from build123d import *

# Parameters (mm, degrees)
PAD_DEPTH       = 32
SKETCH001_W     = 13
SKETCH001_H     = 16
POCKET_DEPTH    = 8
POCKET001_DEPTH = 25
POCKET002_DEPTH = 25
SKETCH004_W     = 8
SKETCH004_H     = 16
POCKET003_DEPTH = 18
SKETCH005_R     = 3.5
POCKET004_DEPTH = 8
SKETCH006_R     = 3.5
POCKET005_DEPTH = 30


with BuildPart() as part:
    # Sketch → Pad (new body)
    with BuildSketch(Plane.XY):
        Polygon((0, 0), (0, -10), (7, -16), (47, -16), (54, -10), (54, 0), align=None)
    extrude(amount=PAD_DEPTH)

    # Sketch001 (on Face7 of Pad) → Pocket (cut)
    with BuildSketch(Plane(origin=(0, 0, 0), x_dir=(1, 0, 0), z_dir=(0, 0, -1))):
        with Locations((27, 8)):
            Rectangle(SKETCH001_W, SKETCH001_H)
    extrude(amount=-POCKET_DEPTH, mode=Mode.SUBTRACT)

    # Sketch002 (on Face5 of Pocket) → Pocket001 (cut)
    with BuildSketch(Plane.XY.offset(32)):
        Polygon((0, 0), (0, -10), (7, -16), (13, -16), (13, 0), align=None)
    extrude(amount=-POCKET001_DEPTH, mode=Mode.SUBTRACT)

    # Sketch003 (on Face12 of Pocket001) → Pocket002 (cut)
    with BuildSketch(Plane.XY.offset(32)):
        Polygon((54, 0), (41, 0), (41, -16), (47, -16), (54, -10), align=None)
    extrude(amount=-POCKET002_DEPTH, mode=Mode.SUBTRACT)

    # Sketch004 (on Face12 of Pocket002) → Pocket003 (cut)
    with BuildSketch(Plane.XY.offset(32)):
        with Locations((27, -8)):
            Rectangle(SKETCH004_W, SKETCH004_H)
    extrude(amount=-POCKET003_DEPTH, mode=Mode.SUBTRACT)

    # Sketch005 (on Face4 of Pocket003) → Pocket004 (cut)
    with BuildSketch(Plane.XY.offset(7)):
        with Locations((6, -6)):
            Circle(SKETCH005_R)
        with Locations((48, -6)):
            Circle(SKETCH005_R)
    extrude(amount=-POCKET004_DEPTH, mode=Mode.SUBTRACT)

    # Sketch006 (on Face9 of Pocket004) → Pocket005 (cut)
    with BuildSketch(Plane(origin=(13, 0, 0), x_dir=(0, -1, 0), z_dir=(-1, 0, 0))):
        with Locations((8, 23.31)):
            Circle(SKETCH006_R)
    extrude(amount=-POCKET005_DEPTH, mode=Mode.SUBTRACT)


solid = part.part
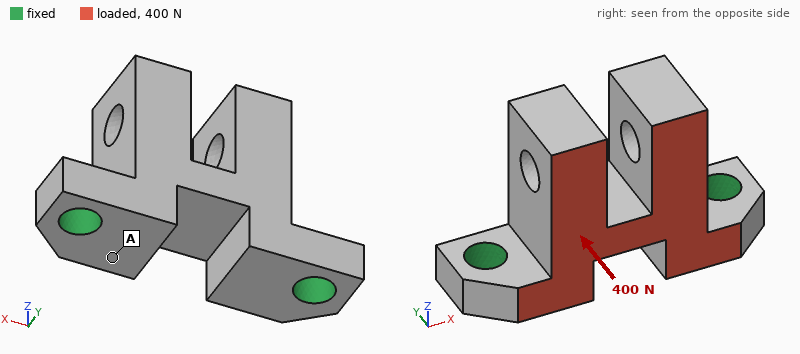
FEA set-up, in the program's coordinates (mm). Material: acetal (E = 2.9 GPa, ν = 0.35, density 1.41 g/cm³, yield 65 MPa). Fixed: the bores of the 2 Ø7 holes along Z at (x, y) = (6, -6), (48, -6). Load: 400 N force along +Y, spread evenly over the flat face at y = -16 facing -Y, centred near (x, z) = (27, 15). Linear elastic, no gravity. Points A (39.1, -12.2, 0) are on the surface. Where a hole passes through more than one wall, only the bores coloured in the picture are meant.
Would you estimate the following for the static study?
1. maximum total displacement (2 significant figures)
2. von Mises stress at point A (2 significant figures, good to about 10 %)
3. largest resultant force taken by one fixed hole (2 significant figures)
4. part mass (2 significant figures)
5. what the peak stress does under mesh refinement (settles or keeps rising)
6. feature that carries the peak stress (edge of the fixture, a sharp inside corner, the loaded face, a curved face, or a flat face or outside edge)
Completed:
0.37 mm
5.1 MPa
200 N
16 g
keeps rising
edge of the fixture
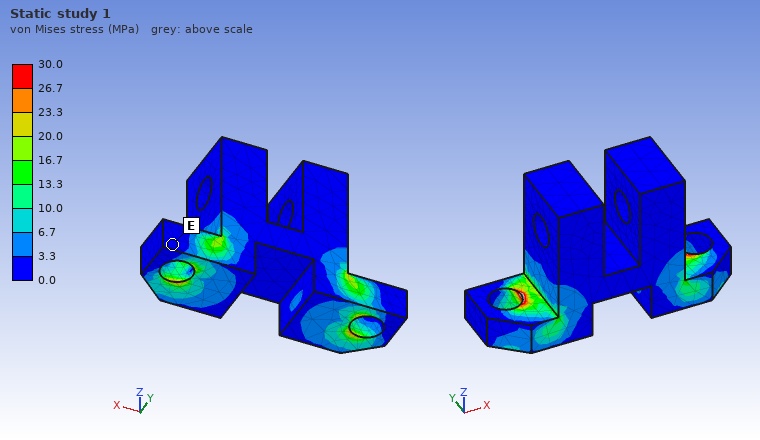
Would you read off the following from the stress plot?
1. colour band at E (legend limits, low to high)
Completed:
0.0 to 3.3 MPa
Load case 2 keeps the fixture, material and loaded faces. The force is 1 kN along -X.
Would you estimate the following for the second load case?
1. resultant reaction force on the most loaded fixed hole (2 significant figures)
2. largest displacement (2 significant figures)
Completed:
630 N
0.36 mm
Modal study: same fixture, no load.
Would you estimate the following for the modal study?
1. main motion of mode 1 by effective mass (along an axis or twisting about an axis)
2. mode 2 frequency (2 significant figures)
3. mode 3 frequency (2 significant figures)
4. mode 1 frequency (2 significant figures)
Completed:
along Y
2800 Hz
3200 Hz
1700 Hz
